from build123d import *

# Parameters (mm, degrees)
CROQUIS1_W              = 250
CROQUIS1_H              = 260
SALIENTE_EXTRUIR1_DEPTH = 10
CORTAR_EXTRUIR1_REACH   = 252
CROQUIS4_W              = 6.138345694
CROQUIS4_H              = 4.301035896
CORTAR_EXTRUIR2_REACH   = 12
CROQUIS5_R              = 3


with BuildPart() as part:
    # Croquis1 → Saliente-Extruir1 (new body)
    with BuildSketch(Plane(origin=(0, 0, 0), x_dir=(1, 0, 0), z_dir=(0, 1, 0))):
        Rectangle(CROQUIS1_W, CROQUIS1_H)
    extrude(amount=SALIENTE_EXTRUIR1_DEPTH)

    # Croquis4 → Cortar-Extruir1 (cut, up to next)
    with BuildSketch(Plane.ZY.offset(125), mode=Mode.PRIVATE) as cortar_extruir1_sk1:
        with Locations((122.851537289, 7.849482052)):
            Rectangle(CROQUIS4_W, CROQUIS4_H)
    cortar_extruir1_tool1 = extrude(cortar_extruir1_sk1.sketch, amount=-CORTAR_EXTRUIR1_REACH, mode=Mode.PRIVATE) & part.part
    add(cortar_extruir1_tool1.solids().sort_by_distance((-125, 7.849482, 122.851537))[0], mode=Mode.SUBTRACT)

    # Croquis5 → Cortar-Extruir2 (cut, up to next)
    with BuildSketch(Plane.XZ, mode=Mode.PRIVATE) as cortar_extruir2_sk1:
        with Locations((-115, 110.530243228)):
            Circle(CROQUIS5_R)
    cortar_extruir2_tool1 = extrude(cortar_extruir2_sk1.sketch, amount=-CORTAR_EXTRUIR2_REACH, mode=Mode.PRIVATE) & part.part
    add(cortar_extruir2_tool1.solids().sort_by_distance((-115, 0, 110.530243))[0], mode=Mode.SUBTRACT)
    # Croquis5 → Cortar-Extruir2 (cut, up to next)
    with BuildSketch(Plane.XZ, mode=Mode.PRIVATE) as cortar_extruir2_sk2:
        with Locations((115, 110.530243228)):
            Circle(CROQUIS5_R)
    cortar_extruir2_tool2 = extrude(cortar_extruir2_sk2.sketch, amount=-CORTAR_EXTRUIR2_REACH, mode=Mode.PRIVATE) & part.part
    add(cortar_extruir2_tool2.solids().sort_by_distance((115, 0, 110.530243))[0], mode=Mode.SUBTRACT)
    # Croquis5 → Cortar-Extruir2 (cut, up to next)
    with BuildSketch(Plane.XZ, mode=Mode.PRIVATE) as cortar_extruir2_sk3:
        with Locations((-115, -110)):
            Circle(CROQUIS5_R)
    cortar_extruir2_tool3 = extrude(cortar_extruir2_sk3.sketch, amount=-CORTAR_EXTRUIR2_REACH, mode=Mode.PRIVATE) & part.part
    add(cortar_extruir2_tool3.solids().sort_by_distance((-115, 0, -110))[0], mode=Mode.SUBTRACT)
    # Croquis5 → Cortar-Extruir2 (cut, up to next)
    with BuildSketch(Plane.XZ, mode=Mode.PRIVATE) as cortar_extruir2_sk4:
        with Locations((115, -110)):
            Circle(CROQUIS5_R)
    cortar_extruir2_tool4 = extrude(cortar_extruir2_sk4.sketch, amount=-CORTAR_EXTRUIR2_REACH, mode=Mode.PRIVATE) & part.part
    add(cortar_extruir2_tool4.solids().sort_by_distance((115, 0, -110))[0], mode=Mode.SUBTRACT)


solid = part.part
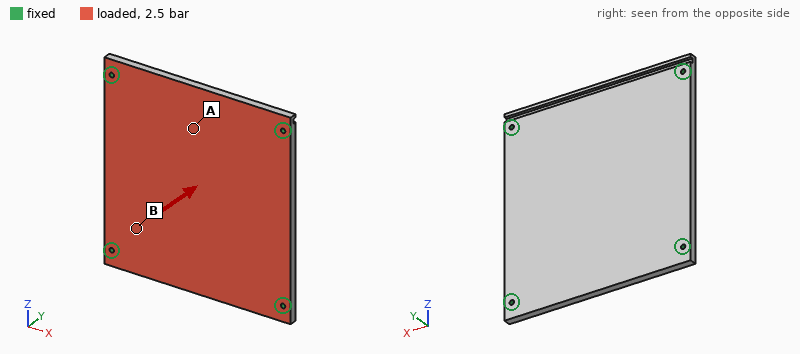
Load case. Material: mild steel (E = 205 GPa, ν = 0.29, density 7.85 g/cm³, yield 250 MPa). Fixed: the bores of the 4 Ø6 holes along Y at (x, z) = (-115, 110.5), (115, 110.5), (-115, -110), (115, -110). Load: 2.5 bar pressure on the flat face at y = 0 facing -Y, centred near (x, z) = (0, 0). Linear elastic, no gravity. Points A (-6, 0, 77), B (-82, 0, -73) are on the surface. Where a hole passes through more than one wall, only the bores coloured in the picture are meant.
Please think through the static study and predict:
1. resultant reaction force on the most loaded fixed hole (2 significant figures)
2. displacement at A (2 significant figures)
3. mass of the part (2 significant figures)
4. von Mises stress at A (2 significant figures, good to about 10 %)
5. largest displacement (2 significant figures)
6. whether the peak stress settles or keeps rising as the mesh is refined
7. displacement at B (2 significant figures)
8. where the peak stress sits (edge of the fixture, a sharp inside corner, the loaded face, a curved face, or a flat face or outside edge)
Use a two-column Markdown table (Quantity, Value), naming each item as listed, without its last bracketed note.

| Quantity | Value |
|---|---|
| resultant reaction force on the most loaded fixed hole | 4.1 kN |
| displacement at A | 0.27 mm |
| mass of the part | 5.0 kg |
| von Mises stress at A | 47 MPa |
| largest displacement | 0.34 mm |
| whether the peak stress settles or keeps rising as the mesh is refined | keeps rising |
| displacement at B | 0.14 mm |
| where the peak stress sits | edge of the fixture |
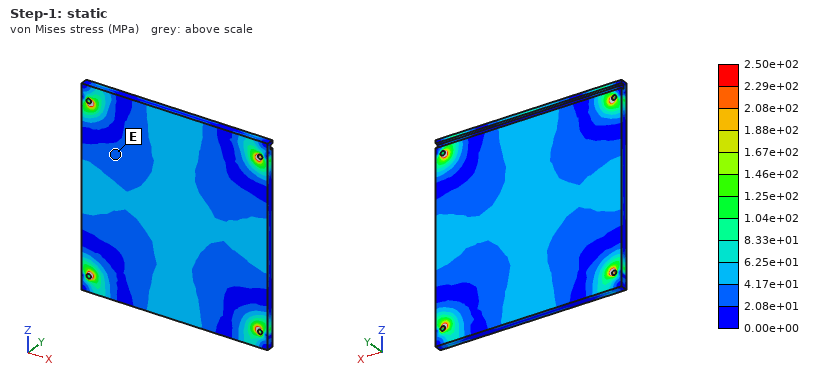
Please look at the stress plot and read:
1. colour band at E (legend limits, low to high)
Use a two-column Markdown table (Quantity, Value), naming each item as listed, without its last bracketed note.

| Quantity | Value |
|---|---|
| colour band at E | 2.08e+01 to 4.17e+01 MPa |
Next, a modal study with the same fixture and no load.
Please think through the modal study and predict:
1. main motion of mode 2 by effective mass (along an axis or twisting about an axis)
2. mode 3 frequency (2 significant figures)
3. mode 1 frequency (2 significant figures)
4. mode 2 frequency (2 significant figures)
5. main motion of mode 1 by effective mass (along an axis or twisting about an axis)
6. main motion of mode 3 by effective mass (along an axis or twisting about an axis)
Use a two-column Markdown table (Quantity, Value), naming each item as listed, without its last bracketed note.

| Quantity | Value |
|---|---|
| main motion of mode 2 by effective mass | twisting about X |
| mode 3 frequency | 1100 Hz |
| mode 1 frequency | 580 Hz |
| mode 2 frequency | 1000 Hz |
| main motion of mode 1 by effective mass | along Y |
| main motion of mode 3 by effective mass | twisting about Z |
